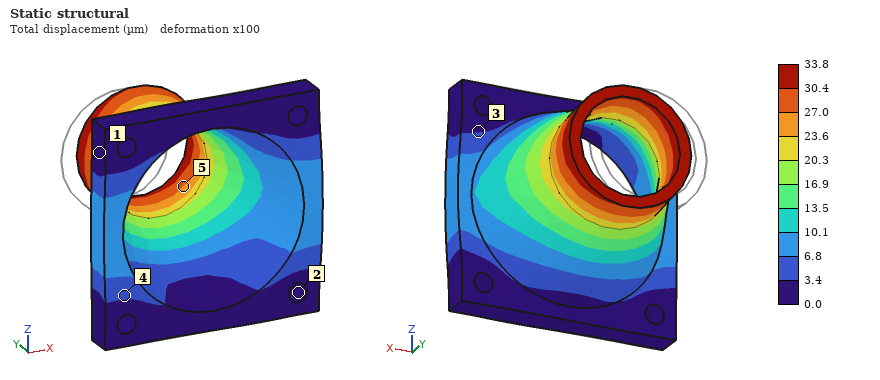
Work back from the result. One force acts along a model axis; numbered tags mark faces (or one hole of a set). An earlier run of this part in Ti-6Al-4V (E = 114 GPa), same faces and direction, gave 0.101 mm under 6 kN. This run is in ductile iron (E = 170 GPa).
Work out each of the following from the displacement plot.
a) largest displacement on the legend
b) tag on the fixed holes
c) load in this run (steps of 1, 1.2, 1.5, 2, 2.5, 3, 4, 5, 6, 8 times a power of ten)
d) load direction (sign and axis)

33.8 µm
2
3 kN
+X
